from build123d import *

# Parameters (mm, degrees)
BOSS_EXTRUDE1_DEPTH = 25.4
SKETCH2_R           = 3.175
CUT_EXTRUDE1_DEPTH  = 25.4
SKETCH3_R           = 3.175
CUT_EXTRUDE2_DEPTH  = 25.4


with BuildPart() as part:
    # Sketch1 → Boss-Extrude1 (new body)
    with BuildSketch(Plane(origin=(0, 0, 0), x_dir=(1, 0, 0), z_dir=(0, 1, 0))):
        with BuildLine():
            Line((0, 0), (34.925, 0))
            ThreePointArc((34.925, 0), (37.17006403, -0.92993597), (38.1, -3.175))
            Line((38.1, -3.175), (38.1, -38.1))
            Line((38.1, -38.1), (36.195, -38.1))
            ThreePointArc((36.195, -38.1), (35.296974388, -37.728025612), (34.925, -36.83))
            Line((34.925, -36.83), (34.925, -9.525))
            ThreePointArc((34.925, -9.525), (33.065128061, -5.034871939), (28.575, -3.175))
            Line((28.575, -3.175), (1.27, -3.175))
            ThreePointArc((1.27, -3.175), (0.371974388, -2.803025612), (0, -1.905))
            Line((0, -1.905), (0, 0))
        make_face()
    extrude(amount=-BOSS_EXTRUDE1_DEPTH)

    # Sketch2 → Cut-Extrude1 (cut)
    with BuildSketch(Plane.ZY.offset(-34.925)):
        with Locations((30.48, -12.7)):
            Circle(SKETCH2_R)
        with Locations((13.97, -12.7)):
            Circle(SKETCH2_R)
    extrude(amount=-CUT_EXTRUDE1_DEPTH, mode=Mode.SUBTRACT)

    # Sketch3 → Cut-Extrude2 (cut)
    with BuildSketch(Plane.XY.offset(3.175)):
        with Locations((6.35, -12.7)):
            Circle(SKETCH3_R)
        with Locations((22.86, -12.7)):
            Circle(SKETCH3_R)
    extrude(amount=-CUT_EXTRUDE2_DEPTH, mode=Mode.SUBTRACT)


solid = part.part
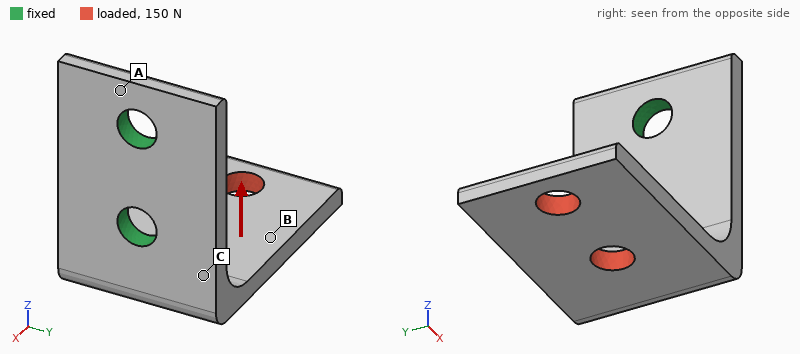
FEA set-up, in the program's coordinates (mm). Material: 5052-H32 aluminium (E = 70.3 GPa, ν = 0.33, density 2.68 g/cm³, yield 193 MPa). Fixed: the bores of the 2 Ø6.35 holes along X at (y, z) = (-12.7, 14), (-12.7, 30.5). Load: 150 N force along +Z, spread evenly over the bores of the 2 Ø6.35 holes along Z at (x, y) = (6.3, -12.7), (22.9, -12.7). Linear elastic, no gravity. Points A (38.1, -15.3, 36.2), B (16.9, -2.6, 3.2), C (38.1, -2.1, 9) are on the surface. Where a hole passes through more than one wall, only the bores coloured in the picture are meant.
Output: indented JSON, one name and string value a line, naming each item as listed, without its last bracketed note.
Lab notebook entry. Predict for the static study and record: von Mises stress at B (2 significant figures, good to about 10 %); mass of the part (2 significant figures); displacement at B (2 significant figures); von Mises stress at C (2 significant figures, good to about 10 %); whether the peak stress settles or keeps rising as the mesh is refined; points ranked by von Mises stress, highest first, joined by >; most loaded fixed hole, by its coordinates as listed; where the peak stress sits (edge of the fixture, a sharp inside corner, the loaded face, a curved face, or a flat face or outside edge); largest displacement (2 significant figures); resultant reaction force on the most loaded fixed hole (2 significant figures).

{
  "von Mises stress at B": "21 MPa",
  "mass of the part": "15 g",
  "displacement at B": "0.14 mm",
  "von Mises stress at C": "55 MPa",
  "whether the peak stress settles or keeps rising as the mesh is refined": "keeps rising",
  "points ranked by von Mises stress, highest first, joined by >": "C > B > A",
  "most loaded fixed hole, by its coordinates as listed": "(-12.7, 14)",
  "where the peak stress sits": "edge of the fixture",
  "largest displacement": "0.34 mm",
  "resultant reaction force on the most loaded fixed hole": "140 N"
}
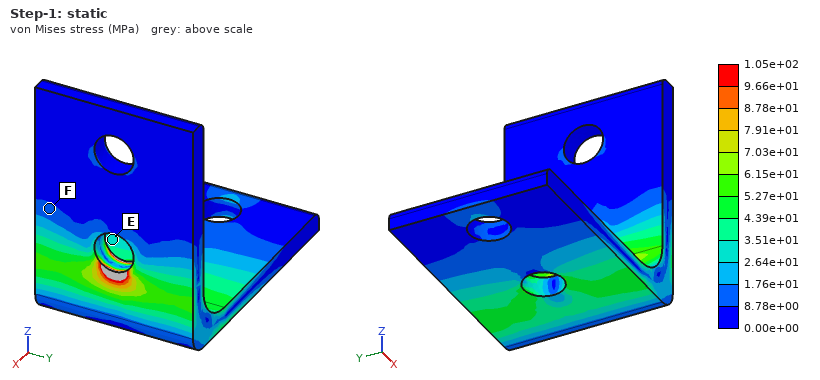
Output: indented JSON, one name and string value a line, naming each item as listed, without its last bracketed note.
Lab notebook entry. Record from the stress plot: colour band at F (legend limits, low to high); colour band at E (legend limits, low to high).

{
  "colour band at F": "8.78e+00 to 1.76e+01 MPa",
  "colour band at E": "2.64e+01 to 3.51e+01 MPa"
}
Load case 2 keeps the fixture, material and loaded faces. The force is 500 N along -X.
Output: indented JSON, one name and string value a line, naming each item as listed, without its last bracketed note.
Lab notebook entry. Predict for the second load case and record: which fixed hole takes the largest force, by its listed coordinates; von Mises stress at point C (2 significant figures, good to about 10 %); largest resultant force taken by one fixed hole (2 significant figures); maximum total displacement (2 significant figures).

{
  "which fixed hole takes the largest force, by its listed coordinates": "(-12.7, 14)",
  "von Mises stress at point C": "53 MPa",
  "largest resultant force taken by one fixed hole": "560 N",
  "maximum total displacement": "0.20 mm"
}
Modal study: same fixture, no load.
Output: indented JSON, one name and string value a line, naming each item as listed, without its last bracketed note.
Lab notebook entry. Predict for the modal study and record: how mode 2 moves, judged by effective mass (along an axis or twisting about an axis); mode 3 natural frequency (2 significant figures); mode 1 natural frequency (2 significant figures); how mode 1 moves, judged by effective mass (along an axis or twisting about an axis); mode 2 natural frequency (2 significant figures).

{
  "how mode 2 moves, judged by effective mass": "along Y",
  "mode 3 natural frequency": "6200 Hz",
  "mode 1 natural frequency": "1700 Hz",
  "how mode 1 moves, judged by effective mass": "along Z",
  "mode 2 natural frequency": "2900 Hz"
}
